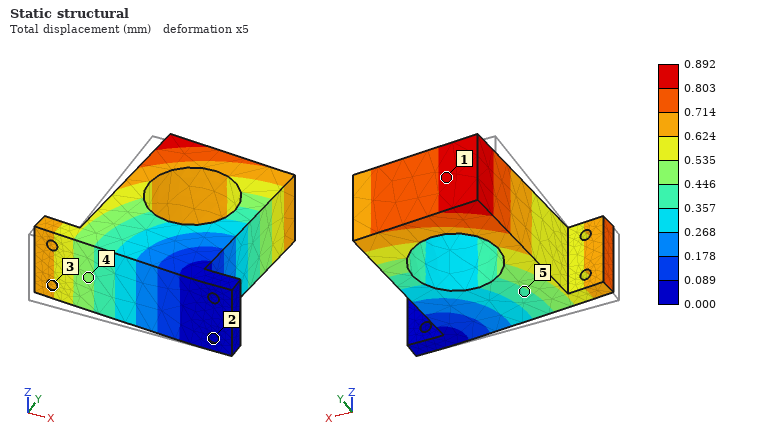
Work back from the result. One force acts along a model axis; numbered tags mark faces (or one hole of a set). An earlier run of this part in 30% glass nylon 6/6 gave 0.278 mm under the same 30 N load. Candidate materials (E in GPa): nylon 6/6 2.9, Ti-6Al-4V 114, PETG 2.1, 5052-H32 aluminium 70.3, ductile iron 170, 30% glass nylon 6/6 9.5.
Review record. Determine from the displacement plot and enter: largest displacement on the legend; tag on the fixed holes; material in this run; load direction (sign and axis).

0.892 mm
2
nylon 6/6
+Y
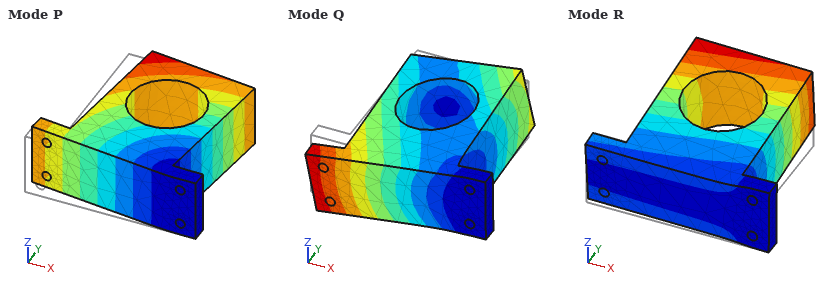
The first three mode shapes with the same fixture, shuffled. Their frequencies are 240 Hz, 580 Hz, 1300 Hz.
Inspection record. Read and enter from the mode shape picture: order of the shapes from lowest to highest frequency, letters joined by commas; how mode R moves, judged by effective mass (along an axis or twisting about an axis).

P, R, Q
along Z
